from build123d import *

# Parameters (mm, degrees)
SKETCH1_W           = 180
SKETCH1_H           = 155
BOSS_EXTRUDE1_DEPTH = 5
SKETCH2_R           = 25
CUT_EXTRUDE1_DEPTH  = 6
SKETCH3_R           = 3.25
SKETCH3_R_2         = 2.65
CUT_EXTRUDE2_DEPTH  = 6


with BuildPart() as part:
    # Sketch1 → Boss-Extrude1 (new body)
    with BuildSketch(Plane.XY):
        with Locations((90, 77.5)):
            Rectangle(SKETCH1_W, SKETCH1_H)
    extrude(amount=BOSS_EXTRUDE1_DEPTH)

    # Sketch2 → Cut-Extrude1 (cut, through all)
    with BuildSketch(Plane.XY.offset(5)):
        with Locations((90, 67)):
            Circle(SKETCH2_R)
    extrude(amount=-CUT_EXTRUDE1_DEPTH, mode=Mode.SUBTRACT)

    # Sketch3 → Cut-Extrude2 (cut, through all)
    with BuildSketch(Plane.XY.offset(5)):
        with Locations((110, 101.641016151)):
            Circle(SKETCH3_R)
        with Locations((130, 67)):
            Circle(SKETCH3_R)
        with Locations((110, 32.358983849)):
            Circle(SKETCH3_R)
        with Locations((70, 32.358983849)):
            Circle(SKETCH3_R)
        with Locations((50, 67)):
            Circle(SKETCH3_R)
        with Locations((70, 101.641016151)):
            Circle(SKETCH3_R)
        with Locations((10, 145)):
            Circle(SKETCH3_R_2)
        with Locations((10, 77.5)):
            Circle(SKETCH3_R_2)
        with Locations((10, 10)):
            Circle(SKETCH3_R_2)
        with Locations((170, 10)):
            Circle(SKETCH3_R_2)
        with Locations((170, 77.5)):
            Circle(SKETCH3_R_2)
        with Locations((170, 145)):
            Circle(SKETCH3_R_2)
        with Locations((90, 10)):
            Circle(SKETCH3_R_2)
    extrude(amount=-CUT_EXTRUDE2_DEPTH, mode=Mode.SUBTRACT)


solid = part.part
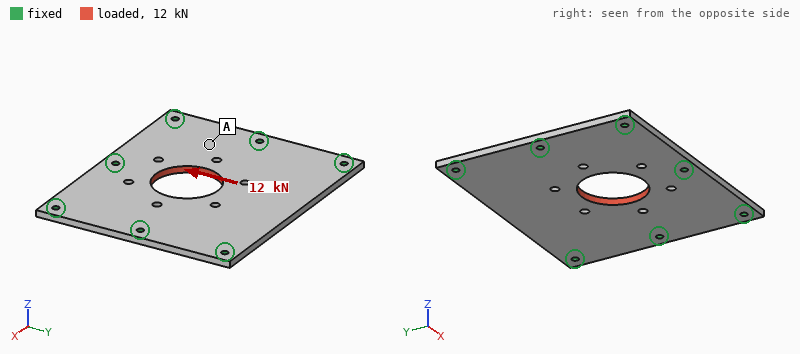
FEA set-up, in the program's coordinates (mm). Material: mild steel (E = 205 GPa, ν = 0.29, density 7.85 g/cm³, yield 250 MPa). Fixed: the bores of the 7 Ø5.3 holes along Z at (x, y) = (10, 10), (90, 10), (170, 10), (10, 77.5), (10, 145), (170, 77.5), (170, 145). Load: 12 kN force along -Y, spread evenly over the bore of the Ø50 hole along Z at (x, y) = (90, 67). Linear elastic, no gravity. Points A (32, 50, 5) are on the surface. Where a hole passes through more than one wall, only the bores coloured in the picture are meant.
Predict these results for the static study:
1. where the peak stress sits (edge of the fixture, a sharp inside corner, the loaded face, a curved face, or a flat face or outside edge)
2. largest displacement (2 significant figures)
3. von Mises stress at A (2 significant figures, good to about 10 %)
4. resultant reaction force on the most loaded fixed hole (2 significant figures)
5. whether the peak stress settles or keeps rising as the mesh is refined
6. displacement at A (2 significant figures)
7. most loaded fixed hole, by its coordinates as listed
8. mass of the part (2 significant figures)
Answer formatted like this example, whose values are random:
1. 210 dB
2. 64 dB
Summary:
1. edge of the fixture
2. 8.3 µm
3. 9.4 MPa
4. 3.7 kN
5. keeps rising
6. 2.4 µm
7. (90, 10)
8. 1.0 kg
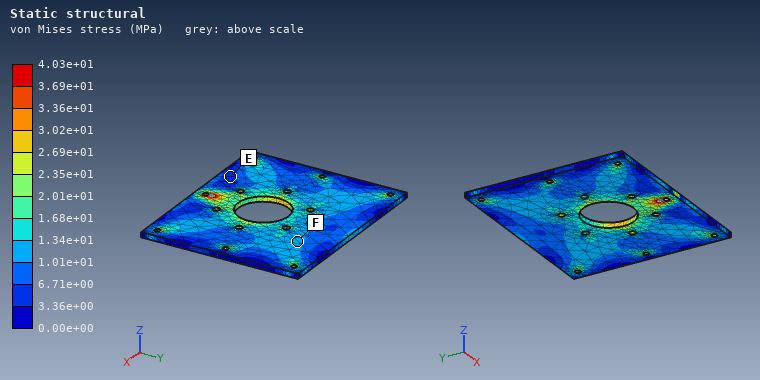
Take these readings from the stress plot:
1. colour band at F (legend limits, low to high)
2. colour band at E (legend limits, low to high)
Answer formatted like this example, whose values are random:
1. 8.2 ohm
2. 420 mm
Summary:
1. 1.01e+01 to 1.34e+01 MPa
2. 3.36e+00 to 6.71e+00 MPa
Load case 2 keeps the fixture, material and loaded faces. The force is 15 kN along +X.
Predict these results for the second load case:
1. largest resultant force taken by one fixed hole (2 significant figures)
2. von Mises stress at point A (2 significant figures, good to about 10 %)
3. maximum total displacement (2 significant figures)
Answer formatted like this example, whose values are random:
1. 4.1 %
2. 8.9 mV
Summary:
1. 3.1 kN
2. 9.2 MPa
3. 6.7 µm
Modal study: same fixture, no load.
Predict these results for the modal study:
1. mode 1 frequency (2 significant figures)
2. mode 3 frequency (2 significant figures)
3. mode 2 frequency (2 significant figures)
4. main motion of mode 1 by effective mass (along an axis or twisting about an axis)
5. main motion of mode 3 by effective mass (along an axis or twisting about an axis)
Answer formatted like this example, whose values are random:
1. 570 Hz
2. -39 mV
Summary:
1. 1000 Hz
2. 2500 Hz
3. 2000 Hz
4. along Z
5. twisting about Y
